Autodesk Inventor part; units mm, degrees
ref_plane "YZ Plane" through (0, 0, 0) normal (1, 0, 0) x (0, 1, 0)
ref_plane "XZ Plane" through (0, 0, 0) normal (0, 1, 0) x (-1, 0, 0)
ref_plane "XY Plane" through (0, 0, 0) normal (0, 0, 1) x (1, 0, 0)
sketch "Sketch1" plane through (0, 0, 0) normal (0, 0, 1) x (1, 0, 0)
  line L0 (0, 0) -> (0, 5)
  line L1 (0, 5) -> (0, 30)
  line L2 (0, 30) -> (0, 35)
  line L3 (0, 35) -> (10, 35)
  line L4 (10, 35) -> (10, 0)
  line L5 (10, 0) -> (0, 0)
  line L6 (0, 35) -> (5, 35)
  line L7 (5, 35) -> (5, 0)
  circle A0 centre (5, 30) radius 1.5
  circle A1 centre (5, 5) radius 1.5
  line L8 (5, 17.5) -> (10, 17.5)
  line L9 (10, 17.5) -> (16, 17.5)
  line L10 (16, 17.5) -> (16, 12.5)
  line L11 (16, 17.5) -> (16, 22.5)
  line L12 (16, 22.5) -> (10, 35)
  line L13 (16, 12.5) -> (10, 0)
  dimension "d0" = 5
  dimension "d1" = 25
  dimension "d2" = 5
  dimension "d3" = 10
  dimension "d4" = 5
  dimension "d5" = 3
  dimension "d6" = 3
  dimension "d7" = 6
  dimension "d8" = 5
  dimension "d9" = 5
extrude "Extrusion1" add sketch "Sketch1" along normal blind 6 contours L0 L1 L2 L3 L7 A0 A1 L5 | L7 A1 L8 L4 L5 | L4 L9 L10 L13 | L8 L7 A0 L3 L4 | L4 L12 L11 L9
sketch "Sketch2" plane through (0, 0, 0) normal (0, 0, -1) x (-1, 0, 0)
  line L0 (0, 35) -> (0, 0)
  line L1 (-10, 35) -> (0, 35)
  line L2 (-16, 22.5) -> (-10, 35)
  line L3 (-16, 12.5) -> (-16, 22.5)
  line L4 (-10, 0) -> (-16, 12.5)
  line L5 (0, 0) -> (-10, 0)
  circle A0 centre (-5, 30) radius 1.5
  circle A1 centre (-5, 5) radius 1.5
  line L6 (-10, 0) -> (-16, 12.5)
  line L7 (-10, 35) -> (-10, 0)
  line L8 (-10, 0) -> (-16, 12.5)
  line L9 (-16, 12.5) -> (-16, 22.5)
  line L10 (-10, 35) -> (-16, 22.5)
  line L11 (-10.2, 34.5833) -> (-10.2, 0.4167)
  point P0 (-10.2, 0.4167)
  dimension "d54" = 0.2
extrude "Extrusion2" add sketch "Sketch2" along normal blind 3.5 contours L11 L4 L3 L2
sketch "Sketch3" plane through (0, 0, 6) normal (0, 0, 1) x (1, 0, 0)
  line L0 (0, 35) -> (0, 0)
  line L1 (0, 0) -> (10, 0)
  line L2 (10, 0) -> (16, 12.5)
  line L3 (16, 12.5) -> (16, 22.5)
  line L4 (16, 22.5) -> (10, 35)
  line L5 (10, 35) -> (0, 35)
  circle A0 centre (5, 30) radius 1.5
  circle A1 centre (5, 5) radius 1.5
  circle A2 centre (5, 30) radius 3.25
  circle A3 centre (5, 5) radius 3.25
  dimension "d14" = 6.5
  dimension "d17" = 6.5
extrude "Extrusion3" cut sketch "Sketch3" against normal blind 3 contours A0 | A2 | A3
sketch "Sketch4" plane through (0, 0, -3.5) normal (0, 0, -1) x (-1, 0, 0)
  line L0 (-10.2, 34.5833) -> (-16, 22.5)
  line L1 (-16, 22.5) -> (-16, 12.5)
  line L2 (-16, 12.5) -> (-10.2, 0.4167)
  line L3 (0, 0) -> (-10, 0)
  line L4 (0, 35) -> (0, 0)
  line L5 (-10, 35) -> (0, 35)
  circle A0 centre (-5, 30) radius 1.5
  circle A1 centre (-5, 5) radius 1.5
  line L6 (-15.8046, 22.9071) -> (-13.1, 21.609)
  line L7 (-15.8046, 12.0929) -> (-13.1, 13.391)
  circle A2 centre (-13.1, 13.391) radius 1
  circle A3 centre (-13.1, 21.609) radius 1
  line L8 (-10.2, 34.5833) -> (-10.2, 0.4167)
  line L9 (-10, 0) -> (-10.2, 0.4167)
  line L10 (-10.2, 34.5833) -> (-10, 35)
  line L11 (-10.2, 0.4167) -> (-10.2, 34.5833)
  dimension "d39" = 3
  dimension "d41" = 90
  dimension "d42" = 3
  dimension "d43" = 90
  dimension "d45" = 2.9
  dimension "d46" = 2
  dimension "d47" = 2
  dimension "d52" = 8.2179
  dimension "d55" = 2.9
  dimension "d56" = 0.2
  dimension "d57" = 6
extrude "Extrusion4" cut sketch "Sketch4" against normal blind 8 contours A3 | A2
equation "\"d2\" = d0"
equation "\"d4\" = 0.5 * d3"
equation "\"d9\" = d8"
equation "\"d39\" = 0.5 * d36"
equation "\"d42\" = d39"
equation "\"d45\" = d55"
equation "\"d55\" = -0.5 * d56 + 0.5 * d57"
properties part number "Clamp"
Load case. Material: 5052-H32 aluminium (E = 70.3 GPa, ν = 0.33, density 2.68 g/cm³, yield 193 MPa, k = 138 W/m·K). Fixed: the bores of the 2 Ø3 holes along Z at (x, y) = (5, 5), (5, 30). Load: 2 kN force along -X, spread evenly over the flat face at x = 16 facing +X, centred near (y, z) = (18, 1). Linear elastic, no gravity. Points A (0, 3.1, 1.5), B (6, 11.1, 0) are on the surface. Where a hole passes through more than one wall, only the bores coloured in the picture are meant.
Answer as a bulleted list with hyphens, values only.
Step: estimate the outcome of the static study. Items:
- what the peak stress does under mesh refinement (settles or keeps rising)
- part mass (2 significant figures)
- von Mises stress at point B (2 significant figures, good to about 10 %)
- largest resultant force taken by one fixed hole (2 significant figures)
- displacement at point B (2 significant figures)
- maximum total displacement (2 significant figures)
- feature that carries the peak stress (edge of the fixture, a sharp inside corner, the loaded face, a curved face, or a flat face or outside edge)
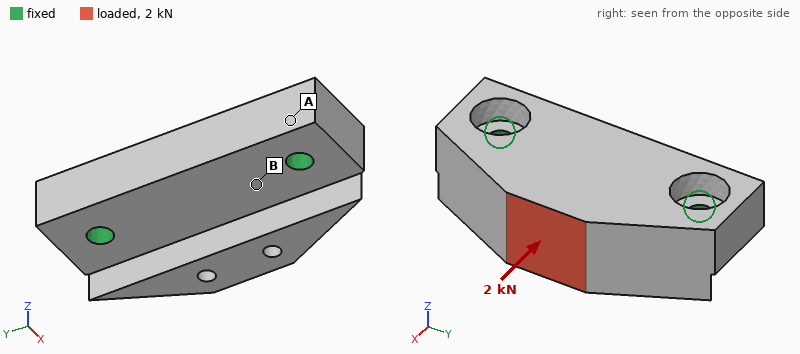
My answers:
- keeps rising
- 8.2 g
- 34 MPa
- 1.1 kN
- 6.1 µm
- 20 µm
- edge of the fixture
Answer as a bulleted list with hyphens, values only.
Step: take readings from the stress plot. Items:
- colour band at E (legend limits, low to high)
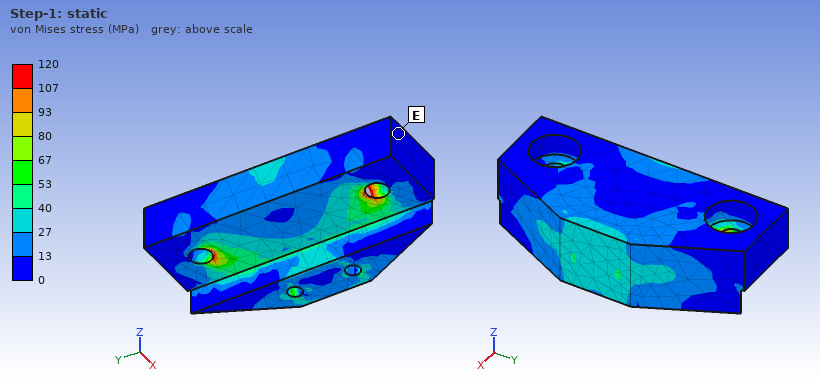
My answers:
- 0 to 13 MPa
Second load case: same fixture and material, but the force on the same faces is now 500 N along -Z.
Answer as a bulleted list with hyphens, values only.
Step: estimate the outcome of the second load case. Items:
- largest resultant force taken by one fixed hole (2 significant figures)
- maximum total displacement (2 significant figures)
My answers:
- 260 N
- 38 µm
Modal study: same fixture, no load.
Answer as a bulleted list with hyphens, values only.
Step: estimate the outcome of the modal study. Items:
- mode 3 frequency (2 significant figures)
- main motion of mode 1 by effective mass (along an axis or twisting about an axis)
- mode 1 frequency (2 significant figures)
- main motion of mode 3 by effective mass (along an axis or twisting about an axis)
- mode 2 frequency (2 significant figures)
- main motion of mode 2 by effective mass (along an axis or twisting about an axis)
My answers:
- 36 kHz
- along Z
- 15 kHz
- along X
- 31 kHz
- along Z
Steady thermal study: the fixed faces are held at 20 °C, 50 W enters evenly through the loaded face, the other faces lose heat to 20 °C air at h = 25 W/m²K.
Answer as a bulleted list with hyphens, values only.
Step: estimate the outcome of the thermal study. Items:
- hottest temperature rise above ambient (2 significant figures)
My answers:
- 51 K
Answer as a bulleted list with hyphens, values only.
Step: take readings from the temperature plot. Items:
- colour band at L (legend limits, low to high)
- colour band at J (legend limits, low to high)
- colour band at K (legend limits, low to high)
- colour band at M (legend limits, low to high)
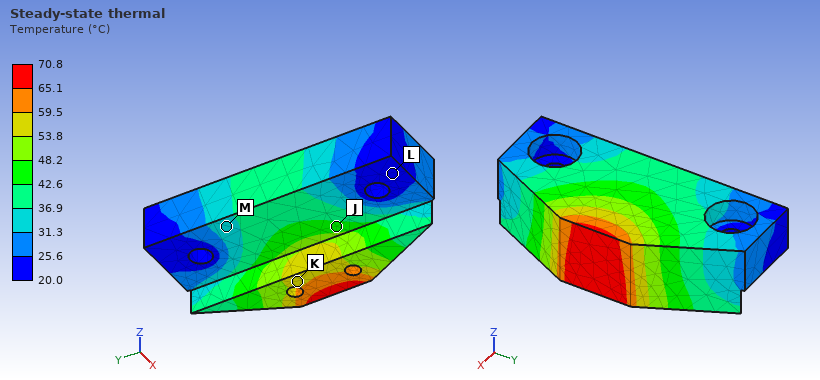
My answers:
- 20.0 to 25.6 °C
- 42.6 to 48.2 °C
- 53.8 to 59.5 °C
- 31.3 to 36.9 °C
